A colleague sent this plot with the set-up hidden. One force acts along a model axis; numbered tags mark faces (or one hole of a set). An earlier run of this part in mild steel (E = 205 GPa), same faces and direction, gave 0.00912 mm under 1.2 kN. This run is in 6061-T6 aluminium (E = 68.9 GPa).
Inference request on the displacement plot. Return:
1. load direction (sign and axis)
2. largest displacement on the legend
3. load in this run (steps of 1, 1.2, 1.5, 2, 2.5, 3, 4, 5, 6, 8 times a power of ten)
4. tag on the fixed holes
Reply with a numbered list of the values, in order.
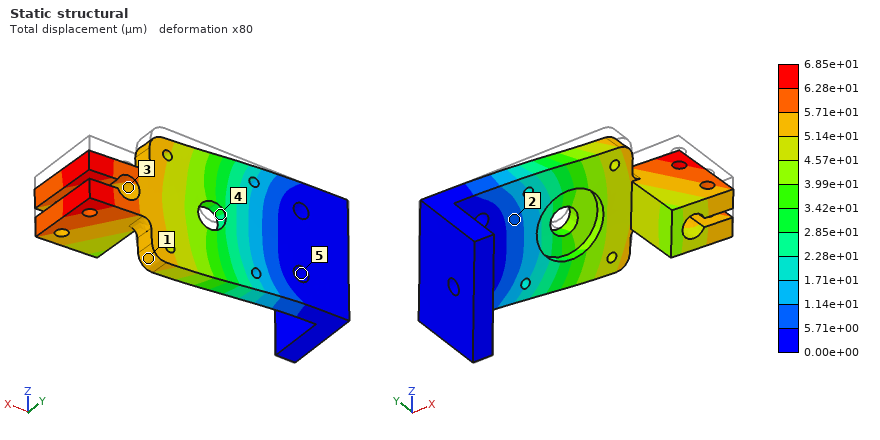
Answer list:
1. -Z
2. 6.85e+01 µm
3. 3 kN
4. 5
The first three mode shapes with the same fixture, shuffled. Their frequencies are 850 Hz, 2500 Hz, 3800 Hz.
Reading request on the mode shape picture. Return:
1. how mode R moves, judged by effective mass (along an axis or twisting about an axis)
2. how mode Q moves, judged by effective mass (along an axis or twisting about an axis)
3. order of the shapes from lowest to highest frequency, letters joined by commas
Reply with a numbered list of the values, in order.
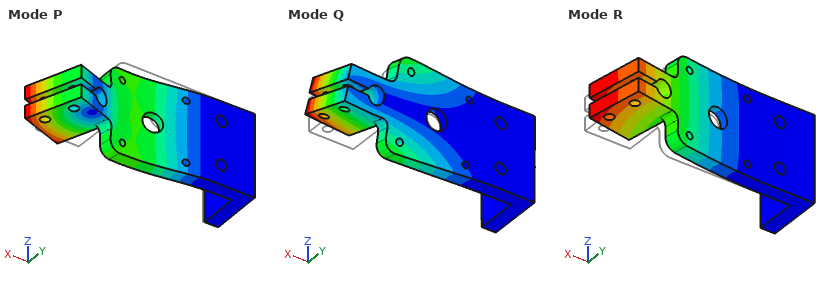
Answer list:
1. along Y
2. along Z
3. R, Q, P
